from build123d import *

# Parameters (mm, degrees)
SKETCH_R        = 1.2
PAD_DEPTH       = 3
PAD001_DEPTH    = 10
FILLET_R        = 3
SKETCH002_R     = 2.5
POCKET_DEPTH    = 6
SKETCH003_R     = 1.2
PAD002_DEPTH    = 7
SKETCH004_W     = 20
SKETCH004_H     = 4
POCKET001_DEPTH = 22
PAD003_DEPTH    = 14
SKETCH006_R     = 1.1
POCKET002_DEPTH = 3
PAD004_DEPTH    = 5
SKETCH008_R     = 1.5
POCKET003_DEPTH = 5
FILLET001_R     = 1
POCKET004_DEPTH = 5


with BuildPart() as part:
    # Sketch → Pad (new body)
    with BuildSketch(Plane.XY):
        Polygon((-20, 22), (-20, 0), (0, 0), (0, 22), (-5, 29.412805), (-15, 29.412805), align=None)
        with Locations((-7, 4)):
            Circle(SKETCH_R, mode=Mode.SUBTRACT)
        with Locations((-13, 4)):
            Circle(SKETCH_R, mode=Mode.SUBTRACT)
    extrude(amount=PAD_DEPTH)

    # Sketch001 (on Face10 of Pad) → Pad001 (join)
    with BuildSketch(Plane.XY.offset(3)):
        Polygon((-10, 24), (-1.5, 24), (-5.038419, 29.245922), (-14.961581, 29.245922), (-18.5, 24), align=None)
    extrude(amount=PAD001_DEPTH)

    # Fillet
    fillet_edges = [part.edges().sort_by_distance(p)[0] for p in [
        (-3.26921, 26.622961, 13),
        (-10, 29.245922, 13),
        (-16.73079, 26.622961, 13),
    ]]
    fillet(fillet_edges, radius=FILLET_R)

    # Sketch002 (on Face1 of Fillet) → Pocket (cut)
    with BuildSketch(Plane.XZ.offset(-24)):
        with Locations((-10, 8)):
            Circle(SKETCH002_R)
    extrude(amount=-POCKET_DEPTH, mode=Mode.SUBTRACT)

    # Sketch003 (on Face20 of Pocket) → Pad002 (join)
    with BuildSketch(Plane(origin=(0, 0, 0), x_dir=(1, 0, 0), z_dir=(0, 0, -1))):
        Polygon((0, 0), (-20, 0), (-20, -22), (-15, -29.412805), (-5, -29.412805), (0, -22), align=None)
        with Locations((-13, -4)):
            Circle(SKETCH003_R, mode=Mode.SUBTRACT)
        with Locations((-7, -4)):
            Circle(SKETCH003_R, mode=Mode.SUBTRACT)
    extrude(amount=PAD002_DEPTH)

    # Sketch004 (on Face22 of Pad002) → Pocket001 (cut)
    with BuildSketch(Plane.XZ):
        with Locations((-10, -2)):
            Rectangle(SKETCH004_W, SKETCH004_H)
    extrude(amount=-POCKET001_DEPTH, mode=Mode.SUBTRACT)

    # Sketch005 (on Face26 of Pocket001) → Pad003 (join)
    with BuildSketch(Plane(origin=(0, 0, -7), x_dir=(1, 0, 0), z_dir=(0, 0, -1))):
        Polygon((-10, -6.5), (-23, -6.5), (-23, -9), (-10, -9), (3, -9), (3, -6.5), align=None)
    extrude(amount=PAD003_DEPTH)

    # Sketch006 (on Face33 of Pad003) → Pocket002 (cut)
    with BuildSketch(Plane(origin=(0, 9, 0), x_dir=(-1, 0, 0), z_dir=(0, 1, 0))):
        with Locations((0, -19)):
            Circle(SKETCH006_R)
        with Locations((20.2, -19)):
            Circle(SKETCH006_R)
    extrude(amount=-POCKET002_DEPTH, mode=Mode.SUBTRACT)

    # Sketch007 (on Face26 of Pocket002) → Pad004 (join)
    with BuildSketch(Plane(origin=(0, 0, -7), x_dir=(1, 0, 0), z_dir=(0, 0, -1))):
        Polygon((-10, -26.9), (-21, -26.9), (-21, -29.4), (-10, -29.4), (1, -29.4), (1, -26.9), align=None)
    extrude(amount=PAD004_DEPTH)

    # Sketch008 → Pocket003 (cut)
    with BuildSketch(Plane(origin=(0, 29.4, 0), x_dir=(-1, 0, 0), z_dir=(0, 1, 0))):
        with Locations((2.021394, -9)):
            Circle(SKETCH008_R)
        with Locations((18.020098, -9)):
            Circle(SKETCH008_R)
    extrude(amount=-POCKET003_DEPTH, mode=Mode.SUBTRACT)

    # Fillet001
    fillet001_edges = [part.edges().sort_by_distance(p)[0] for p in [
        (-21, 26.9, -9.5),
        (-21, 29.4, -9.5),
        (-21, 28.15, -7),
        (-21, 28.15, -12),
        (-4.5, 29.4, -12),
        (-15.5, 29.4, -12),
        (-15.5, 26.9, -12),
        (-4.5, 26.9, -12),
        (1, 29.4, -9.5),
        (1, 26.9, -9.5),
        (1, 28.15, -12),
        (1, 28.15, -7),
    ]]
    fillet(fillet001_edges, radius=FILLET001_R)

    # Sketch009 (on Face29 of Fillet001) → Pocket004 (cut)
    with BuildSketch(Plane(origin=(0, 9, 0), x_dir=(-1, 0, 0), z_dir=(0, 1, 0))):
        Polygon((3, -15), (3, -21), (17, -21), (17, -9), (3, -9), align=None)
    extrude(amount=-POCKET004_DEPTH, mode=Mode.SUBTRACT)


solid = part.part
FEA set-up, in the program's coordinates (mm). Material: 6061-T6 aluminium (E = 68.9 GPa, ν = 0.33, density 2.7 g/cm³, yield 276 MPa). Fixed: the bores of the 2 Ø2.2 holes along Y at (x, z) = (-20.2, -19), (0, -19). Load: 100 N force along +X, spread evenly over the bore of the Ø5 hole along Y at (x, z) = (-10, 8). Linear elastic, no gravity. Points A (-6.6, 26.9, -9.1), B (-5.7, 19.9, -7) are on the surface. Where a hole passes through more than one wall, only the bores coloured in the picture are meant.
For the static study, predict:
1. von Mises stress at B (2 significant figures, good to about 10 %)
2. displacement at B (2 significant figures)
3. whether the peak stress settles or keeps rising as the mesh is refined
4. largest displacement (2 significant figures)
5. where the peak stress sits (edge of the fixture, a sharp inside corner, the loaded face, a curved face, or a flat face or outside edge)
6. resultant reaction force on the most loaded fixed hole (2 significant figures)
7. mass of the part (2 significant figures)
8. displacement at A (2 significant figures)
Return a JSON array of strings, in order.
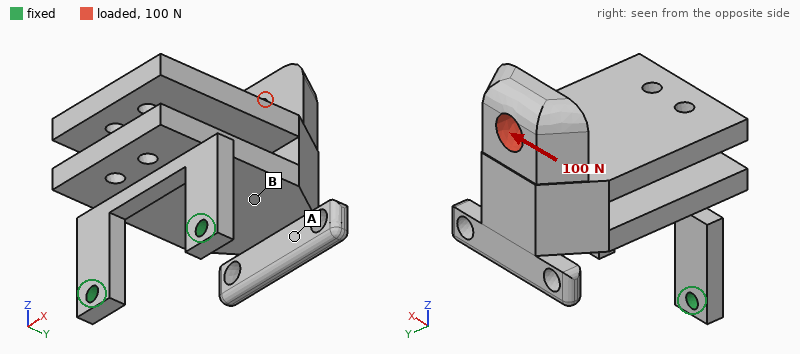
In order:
["19 MPa", "0.047 mm", "keeps rising", "0.11 mm", "edge of the fixture", "140 N", "13 g", "0.063 mm"]
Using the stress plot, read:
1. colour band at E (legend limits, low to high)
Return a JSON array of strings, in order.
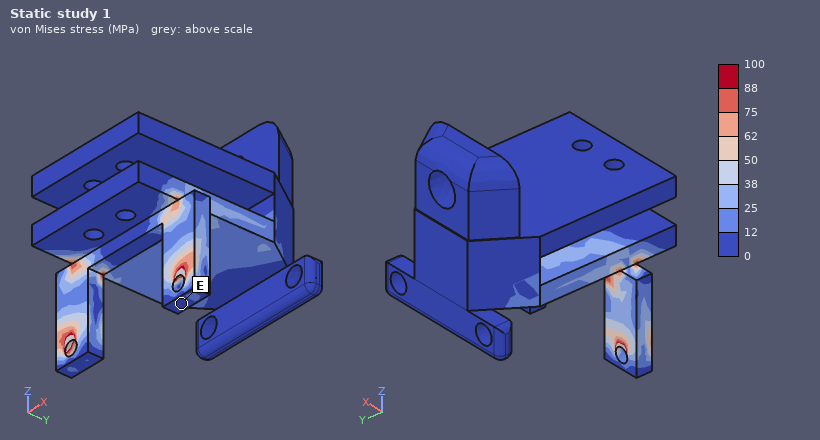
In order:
["0 to 12 MPa"]
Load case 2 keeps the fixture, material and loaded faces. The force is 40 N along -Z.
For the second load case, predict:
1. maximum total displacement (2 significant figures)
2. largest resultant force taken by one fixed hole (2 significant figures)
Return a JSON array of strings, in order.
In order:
["0.35 mm", "21 N"]
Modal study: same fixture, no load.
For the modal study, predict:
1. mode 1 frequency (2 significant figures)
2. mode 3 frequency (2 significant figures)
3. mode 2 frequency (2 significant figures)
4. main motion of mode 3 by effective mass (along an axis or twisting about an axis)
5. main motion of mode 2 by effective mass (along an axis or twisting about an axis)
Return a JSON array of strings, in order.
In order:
["680 Hz", "3100 Hz", "2200 Hz", "along Z", "along X"]
